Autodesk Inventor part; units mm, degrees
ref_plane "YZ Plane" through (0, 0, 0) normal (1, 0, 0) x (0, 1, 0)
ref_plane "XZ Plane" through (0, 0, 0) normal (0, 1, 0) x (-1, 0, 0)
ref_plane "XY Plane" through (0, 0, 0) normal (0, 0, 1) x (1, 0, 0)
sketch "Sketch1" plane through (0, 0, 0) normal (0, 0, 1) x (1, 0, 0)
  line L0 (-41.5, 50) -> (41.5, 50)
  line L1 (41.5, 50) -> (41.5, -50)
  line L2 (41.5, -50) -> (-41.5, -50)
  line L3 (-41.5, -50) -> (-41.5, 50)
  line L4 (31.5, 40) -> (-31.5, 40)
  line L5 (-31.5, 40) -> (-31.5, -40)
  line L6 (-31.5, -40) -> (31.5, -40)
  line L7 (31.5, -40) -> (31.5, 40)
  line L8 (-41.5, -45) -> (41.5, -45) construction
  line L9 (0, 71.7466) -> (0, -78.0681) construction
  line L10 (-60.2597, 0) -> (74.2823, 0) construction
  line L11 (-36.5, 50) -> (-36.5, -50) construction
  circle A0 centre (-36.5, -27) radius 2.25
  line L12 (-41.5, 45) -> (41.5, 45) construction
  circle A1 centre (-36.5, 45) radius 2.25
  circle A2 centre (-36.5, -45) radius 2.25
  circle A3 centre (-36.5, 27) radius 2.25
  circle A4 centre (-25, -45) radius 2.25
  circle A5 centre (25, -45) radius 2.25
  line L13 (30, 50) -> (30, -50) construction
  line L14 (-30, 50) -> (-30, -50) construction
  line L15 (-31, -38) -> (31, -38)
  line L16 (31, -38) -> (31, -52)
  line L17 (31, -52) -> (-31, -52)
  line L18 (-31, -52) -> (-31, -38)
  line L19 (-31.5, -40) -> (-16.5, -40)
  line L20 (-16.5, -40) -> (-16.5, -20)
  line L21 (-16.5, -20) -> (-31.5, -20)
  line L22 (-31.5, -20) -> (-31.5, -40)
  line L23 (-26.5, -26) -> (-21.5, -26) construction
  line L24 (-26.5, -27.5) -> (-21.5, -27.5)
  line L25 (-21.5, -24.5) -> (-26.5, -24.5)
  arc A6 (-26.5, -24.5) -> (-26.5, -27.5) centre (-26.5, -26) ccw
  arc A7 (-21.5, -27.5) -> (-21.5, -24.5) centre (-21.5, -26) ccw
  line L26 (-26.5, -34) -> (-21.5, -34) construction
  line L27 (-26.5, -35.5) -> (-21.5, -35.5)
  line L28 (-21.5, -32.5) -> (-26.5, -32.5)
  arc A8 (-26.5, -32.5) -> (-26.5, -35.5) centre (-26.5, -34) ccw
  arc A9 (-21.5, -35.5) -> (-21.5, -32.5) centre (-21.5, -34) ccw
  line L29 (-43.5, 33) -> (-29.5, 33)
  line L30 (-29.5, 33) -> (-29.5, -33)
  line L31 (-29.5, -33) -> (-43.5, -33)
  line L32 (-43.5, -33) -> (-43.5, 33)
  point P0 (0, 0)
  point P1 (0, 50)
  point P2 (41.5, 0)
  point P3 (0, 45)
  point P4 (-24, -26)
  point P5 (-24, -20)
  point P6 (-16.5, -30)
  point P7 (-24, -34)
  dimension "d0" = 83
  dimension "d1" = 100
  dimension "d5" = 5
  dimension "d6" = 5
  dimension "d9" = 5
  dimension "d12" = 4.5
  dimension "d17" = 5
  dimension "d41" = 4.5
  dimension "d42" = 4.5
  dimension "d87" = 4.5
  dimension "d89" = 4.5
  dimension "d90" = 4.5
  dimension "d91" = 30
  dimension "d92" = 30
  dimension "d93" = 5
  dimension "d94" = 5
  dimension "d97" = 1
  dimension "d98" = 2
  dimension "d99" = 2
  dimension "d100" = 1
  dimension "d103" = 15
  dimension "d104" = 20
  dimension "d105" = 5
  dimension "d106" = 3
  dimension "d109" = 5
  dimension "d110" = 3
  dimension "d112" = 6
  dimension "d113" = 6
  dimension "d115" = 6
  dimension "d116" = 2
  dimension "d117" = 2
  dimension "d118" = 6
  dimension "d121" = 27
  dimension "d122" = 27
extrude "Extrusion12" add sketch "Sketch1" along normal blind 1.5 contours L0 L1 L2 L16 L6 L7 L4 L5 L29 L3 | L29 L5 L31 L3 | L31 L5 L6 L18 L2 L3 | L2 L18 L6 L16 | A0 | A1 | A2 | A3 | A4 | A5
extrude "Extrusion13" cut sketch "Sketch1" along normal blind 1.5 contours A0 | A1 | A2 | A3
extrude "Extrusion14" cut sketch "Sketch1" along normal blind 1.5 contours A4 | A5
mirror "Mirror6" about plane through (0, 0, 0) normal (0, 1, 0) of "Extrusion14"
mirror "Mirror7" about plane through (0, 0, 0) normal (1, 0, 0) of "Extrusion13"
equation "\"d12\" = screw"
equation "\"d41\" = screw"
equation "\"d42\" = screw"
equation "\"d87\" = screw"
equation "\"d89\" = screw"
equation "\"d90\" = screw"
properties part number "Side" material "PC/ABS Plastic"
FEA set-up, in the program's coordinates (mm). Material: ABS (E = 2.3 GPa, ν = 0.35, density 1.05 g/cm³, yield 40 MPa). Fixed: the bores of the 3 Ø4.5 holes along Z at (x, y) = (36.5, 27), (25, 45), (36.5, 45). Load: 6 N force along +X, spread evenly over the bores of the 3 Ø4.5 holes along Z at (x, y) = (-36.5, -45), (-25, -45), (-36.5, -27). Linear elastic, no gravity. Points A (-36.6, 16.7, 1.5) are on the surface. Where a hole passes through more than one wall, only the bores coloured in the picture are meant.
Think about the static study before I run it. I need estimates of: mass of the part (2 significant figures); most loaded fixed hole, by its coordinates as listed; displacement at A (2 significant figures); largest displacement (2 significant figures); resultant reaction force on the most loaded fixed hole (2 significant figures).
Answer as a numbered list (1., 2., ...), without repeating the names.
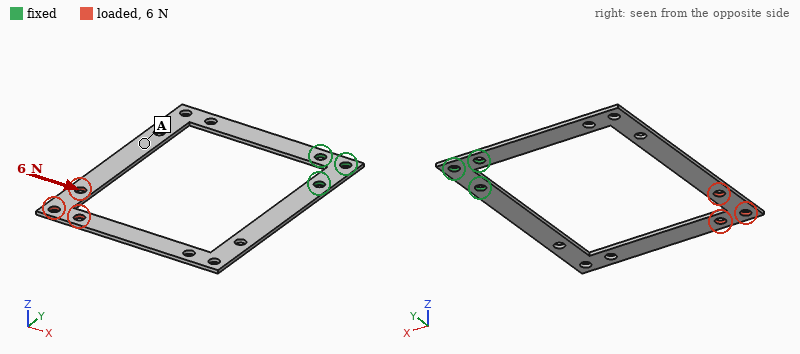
1. 4.8 g
2. (36.5, 27)
3. 0.84 mm
4. 1.5 mm
5. 9.2 N
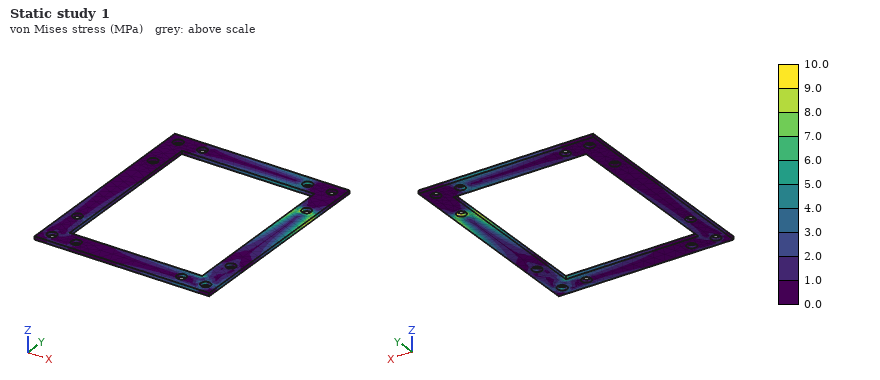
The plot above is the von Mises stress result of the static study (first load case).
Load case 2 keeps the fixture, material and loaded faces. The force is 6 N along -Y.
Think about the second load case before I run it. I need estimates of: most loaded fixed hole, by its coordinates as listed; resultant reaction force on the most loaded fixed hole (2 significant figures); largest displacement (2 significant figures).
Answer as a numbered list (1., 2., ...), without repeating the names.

1. (25, 45)
2. 10 N
3. 1.2 mm
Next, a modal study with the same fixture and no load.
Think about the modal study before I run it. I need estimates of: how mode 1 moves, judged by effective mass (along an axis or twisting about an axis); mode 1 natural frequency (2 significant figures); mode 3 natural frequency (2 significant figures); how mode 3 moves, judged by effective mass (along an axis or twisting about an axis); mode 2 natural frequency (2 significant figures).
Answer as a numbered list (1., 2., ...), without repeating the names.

1. along Z
2. 25 Hz
3. 100 Hz
4. along Z
5. 55 Hz
